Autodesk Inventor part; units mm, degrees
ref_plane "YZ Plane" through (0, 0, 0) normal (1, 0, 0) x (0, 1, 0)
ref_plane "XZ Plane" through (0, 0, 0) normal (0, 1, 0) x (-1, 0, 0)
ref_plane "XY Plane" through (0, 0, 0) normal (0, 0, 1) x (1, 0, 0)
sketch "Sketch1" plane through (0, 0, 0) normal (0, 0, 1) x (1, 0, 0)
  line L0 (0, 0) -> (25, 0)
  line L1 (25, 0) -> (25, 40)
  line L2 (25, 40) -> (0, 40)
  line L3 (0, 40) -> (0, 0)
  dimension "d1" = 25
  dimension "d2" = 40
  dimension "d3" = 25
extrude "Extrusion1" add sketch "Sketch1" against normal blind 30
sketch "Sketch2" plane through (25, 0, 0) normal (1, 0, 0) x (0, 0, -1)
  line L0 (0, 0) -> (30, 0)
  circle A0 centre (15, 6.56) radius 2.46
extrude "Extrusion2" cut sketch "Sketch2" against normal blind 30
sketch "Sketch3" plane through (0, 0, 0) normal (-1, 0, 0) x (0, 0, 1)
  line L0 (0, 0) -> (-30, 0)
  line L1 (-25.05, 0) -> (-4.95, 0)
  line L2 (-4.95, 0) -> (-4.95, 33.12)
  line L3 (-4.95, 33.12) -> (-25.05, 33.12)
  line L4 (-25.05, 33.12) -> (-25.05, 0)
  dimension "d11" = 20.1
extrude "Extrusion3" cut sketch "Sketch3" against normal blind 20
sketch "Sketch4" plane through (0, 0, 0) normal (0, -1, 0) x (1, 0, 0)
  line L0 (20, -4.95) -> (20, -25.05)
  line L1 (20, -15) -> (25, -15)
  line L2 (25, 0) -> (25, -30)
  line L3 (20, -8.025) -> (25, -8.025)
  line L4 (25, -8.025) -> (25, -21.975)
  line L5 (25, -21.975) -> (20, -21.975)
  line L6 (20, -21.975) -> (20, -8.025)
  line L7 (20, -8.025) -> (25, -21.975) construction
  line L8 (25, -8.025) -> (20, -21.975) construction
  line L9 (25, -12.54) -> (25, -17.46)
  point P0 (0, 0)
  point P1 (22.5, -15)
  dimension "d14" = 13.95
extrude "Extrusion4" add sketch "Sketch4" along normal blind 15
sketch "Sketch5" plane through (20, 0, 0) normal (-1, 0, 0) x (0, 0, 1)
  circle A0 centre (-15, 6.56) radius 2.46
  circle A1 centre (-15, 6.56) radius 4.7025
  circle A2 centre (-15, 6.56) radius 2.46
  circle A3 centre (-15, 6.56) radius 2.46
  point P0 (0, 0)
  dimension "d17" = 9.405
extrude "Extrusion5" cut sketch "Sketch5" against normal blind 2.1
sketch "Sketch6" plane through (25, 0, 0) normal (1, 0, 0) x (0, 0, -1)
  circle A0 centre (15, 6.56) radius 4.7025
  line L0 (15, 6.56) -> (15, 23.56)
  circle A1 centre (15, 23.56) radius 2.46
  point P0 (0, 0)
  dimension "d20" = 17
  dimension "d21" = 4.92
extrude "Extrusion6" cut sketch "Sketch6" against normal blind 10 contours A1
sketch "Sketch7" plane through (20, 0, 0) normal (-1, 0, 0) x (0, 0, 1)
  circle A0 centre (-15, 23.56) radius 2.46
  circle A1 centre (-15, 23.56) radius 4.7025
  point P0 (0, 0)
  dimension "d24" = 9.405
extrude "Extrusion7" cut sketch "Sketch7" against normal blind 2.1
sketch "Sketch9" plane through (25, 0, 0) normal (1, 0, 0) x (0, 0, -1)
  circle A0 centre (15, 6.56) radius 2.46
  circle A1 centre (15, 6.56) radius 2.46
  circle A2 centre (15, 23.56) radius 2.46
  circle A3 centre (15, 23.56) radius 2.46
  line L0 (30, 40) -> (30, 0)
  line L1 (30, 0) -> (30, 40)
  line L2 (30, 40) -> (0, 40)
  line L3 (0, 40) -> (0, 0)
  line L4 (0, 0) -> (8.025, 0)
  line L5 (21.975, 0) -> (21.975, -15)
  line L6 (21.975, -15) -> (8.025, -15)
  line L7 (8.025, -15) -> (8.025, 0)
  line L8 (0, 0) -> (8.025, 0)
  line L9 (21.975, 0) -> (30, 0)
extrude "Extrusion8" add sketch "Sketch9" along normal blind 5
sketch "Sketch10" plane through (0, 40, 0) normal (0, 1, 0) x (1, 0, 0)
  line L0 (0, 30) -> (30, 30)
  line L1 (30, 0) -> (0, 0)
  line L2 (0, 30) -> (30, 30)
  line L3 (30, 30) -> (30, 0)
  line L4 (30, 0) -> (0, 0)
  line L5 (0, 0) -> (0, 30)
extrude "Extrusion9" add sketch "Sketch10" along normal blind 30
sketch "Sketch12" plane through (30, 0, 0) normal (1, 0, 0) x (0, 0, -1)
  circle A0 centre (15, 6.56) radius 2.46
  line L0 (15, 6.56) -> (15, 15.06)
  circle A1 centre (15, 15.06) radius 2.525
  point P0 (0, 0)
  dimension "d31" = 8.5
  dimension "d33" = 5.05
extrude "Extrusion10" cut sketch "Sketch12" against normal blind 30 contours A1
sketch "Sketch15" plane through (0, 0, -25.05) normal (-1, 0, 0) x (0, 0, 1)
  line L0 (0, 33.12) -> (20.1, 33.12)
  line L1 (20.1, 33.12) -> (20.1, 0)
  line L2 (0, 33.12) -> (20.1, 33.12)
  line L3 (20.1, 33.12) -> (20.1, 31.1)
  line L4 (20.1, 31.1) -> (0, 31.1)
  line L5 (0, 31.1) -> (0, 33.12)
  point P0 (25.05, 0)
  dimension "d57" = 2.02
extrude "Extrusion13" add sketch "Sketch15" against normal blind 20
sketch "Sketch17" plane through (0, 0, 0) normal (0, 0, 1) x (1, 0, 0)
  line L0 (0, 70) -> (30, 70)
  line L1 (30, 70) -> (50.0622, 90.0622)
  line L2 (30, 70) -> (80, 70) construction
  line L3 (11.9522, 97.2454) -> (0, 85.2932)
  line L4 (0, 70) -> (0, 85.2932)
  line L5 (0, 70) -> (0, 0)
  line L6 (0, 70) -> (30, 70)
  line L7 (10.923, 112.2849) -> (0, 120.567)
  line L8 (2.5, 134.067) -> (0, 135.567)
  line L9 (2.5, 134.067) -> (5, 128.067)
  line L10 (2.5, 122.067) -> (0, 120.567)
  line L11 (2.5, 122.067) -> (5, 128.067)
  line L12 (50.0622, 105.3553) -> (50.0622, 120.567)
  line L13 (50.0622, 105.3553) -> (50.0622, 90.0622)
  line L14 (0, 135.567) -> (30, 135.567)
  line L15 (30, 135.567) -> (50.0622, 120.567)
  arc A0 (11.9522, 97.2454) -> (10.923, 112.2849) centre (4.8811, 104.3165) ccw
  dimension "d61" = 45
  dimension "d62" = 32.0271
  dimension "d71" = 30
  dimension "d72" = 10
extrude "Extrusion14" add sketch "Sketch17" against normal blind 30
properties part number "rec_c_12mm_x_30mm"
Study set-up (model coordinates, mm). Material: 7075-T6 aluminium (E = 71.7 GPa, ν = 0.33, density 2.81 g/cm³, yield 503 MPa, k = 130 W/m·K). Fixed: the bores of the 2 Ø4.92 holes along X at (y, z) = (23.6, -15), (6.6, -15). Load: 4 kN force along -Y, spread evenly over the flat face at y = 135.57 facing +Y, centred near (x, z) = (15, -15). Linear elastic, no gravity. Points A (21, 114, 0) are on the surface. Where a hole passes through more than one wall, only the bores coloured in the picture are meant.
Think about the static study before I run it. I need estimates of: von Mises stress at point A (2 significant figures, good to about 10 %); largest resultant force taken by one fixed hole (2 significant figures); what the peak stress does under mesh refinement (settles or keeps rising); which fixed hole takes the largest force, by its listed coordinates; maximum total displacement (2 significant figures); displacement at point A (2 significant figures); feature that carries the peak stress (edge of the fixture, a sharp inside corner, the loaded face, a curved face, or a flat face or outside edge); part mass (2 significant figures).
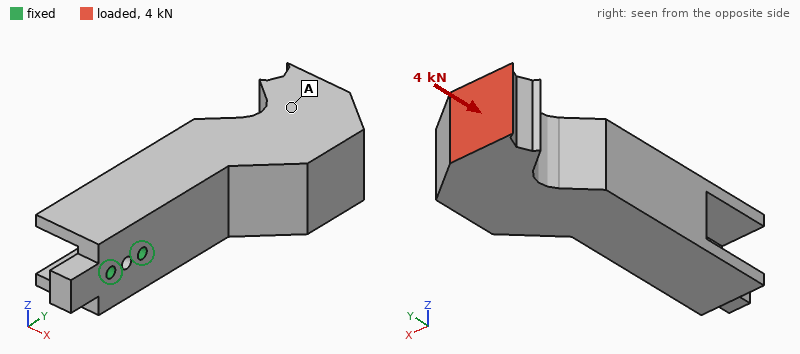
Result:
7.7 MPa
3.0 kN
keeps rising
(23.6, -15)
0.12 mm
0.084 mm
edge of the fixture
360 g
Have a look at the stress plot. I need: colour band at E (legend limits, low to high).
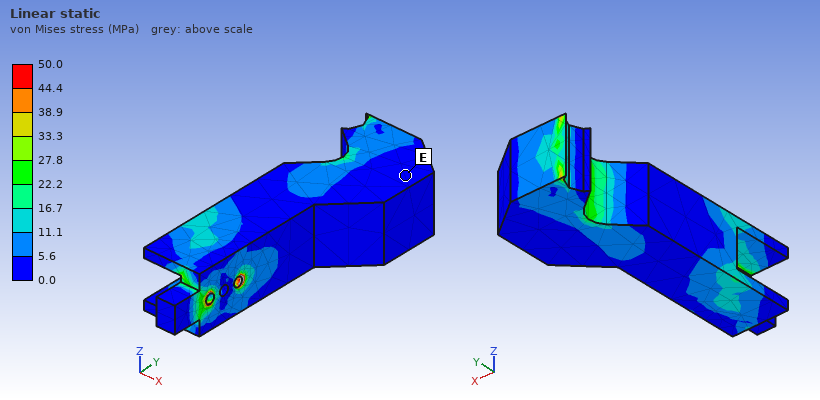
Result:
0.0 to 5.6 MPa
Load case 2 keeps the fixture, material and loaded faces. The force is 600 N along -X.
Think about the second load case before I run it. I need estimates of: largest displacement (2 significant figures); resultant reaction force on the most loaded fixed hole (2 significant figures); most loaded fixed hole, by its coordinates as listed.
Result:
0.22 mm
3.3 kN
(23.6, -15)
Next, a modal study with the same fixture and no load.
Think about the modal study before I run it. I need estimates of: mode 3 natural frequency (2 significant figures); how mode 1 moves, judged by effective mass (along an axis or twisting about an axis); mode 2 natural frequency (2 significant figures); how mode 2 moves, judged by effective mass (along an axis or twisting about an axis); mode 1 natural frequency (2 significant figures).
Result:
2400 Hz
along X
910 Hz
along Z
790 Hz
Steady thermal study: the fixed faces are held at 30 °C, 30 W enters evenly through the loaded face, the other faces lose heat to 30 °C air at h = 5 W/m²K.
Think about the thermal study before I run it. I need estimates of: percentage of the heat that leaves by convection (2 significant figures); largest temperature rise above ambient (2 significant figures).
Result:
5.8 %
38 K
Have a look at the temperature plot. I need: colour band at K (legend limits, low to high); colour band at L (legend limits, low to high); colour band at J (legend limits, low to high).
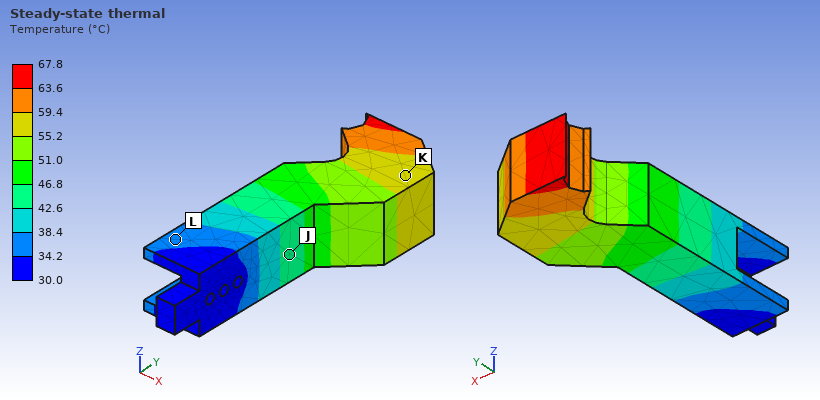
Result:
55.2 to 59.4 °C
34.2 to 38.4 °C
42.6 to 46.8 °C
